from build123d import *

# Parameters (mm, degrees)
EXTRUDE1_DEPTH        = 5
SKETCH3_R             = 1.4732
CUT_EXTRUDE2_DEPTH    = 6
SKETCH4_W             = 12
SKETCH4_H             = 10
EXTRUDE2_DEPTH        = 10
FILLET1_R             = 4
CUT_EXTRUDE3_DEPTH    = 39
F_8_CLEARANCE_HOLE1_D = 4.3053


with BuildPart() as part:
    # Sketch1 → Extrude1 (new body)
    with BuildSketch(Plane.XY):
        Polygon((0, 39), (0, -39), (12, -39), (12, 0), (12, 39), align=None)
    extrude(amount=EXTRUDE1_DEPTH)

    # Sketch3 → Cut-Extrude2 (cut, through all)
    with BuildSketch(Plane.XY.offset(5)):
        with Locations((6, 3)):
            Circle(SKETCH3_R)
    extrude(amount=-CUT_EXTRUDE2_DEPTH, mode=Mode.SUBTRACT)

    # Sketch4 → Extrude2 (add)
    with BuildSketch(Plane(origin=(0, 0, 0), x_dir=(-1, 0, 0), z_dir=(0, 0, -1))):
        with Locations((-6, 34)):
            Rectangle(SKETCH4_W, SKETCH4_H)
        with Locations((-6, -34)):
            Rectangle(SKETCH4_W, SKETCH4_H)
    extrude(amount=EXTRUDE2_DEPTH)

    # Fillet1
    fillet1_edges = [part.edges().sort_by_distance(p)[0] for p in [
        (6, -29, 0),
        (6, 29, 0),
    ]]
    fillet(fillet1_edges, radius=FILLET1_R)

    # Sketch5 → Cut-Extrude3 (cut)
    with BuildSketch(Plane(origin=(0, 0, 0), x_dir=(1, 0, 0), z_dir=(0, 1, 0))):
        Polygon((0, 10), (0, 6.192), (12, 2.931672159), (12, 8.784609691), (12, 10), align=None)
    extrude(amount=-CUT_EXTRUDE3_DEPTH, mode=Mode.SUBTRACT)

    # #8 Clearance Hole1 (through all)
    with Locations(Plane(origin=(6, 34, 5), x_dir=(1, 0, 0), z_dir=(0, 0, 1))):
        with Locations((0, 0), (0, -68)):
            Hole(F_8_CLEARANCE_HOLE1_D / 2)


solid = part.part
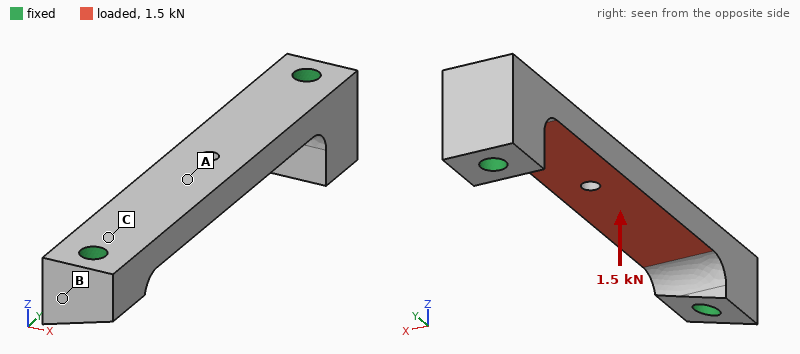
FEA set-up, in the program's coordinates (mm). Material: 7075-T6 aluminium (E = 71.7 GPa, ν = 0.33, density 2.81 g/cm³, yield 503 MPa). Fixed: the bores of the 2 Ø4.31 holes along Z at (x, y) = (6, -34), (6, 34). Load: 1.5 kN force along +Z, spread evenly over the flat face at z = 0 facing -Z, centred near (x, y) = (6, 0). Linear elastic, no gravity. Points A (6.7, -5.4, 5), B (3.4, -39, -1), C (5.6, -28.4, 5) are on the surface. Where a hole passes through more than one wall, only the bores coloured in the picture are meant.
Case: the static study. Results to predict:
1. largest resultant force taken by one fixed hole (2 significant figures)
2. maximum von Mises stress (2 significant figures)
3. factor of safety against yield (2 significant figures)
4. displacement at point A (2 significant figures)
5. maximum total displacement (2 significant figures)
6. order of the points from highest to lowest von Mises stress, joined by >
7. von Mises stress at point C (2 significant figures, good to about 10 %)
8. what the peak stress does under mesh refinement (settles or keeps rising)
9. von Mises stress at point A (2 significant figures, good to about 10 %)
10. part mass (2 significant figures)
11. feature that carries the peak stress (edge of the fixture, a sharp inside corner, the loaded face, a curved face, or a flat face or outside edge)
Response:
800 N
200 MPa
2.6
0.11 mm
0.12 mm
C > A > B
99 MPa
settles
78 MPa
17 g
a curved face
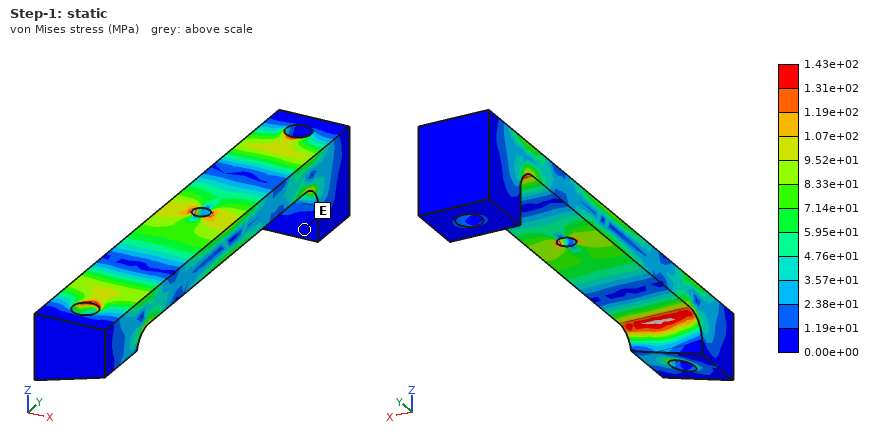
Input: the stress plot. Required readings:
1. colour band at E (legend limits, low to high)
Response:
0.00e+00 to 1.19e+01 MPa
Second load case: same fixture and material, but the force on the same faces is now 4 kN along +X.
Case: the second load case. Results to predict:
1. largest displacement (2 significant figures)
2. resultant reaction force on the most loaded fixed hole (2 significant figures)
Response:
0.15 mm
2.0 kN
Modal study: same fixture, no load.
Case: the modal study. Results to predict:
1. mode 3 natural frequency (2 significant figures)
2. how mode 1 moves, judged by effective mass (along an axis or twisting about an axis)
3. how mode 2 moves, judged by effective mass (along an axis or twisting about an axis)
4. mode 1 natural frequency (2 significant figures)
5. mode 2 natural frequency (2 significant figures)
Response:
18 kHz
along Z
along X
7100 Hz
11 kHz
